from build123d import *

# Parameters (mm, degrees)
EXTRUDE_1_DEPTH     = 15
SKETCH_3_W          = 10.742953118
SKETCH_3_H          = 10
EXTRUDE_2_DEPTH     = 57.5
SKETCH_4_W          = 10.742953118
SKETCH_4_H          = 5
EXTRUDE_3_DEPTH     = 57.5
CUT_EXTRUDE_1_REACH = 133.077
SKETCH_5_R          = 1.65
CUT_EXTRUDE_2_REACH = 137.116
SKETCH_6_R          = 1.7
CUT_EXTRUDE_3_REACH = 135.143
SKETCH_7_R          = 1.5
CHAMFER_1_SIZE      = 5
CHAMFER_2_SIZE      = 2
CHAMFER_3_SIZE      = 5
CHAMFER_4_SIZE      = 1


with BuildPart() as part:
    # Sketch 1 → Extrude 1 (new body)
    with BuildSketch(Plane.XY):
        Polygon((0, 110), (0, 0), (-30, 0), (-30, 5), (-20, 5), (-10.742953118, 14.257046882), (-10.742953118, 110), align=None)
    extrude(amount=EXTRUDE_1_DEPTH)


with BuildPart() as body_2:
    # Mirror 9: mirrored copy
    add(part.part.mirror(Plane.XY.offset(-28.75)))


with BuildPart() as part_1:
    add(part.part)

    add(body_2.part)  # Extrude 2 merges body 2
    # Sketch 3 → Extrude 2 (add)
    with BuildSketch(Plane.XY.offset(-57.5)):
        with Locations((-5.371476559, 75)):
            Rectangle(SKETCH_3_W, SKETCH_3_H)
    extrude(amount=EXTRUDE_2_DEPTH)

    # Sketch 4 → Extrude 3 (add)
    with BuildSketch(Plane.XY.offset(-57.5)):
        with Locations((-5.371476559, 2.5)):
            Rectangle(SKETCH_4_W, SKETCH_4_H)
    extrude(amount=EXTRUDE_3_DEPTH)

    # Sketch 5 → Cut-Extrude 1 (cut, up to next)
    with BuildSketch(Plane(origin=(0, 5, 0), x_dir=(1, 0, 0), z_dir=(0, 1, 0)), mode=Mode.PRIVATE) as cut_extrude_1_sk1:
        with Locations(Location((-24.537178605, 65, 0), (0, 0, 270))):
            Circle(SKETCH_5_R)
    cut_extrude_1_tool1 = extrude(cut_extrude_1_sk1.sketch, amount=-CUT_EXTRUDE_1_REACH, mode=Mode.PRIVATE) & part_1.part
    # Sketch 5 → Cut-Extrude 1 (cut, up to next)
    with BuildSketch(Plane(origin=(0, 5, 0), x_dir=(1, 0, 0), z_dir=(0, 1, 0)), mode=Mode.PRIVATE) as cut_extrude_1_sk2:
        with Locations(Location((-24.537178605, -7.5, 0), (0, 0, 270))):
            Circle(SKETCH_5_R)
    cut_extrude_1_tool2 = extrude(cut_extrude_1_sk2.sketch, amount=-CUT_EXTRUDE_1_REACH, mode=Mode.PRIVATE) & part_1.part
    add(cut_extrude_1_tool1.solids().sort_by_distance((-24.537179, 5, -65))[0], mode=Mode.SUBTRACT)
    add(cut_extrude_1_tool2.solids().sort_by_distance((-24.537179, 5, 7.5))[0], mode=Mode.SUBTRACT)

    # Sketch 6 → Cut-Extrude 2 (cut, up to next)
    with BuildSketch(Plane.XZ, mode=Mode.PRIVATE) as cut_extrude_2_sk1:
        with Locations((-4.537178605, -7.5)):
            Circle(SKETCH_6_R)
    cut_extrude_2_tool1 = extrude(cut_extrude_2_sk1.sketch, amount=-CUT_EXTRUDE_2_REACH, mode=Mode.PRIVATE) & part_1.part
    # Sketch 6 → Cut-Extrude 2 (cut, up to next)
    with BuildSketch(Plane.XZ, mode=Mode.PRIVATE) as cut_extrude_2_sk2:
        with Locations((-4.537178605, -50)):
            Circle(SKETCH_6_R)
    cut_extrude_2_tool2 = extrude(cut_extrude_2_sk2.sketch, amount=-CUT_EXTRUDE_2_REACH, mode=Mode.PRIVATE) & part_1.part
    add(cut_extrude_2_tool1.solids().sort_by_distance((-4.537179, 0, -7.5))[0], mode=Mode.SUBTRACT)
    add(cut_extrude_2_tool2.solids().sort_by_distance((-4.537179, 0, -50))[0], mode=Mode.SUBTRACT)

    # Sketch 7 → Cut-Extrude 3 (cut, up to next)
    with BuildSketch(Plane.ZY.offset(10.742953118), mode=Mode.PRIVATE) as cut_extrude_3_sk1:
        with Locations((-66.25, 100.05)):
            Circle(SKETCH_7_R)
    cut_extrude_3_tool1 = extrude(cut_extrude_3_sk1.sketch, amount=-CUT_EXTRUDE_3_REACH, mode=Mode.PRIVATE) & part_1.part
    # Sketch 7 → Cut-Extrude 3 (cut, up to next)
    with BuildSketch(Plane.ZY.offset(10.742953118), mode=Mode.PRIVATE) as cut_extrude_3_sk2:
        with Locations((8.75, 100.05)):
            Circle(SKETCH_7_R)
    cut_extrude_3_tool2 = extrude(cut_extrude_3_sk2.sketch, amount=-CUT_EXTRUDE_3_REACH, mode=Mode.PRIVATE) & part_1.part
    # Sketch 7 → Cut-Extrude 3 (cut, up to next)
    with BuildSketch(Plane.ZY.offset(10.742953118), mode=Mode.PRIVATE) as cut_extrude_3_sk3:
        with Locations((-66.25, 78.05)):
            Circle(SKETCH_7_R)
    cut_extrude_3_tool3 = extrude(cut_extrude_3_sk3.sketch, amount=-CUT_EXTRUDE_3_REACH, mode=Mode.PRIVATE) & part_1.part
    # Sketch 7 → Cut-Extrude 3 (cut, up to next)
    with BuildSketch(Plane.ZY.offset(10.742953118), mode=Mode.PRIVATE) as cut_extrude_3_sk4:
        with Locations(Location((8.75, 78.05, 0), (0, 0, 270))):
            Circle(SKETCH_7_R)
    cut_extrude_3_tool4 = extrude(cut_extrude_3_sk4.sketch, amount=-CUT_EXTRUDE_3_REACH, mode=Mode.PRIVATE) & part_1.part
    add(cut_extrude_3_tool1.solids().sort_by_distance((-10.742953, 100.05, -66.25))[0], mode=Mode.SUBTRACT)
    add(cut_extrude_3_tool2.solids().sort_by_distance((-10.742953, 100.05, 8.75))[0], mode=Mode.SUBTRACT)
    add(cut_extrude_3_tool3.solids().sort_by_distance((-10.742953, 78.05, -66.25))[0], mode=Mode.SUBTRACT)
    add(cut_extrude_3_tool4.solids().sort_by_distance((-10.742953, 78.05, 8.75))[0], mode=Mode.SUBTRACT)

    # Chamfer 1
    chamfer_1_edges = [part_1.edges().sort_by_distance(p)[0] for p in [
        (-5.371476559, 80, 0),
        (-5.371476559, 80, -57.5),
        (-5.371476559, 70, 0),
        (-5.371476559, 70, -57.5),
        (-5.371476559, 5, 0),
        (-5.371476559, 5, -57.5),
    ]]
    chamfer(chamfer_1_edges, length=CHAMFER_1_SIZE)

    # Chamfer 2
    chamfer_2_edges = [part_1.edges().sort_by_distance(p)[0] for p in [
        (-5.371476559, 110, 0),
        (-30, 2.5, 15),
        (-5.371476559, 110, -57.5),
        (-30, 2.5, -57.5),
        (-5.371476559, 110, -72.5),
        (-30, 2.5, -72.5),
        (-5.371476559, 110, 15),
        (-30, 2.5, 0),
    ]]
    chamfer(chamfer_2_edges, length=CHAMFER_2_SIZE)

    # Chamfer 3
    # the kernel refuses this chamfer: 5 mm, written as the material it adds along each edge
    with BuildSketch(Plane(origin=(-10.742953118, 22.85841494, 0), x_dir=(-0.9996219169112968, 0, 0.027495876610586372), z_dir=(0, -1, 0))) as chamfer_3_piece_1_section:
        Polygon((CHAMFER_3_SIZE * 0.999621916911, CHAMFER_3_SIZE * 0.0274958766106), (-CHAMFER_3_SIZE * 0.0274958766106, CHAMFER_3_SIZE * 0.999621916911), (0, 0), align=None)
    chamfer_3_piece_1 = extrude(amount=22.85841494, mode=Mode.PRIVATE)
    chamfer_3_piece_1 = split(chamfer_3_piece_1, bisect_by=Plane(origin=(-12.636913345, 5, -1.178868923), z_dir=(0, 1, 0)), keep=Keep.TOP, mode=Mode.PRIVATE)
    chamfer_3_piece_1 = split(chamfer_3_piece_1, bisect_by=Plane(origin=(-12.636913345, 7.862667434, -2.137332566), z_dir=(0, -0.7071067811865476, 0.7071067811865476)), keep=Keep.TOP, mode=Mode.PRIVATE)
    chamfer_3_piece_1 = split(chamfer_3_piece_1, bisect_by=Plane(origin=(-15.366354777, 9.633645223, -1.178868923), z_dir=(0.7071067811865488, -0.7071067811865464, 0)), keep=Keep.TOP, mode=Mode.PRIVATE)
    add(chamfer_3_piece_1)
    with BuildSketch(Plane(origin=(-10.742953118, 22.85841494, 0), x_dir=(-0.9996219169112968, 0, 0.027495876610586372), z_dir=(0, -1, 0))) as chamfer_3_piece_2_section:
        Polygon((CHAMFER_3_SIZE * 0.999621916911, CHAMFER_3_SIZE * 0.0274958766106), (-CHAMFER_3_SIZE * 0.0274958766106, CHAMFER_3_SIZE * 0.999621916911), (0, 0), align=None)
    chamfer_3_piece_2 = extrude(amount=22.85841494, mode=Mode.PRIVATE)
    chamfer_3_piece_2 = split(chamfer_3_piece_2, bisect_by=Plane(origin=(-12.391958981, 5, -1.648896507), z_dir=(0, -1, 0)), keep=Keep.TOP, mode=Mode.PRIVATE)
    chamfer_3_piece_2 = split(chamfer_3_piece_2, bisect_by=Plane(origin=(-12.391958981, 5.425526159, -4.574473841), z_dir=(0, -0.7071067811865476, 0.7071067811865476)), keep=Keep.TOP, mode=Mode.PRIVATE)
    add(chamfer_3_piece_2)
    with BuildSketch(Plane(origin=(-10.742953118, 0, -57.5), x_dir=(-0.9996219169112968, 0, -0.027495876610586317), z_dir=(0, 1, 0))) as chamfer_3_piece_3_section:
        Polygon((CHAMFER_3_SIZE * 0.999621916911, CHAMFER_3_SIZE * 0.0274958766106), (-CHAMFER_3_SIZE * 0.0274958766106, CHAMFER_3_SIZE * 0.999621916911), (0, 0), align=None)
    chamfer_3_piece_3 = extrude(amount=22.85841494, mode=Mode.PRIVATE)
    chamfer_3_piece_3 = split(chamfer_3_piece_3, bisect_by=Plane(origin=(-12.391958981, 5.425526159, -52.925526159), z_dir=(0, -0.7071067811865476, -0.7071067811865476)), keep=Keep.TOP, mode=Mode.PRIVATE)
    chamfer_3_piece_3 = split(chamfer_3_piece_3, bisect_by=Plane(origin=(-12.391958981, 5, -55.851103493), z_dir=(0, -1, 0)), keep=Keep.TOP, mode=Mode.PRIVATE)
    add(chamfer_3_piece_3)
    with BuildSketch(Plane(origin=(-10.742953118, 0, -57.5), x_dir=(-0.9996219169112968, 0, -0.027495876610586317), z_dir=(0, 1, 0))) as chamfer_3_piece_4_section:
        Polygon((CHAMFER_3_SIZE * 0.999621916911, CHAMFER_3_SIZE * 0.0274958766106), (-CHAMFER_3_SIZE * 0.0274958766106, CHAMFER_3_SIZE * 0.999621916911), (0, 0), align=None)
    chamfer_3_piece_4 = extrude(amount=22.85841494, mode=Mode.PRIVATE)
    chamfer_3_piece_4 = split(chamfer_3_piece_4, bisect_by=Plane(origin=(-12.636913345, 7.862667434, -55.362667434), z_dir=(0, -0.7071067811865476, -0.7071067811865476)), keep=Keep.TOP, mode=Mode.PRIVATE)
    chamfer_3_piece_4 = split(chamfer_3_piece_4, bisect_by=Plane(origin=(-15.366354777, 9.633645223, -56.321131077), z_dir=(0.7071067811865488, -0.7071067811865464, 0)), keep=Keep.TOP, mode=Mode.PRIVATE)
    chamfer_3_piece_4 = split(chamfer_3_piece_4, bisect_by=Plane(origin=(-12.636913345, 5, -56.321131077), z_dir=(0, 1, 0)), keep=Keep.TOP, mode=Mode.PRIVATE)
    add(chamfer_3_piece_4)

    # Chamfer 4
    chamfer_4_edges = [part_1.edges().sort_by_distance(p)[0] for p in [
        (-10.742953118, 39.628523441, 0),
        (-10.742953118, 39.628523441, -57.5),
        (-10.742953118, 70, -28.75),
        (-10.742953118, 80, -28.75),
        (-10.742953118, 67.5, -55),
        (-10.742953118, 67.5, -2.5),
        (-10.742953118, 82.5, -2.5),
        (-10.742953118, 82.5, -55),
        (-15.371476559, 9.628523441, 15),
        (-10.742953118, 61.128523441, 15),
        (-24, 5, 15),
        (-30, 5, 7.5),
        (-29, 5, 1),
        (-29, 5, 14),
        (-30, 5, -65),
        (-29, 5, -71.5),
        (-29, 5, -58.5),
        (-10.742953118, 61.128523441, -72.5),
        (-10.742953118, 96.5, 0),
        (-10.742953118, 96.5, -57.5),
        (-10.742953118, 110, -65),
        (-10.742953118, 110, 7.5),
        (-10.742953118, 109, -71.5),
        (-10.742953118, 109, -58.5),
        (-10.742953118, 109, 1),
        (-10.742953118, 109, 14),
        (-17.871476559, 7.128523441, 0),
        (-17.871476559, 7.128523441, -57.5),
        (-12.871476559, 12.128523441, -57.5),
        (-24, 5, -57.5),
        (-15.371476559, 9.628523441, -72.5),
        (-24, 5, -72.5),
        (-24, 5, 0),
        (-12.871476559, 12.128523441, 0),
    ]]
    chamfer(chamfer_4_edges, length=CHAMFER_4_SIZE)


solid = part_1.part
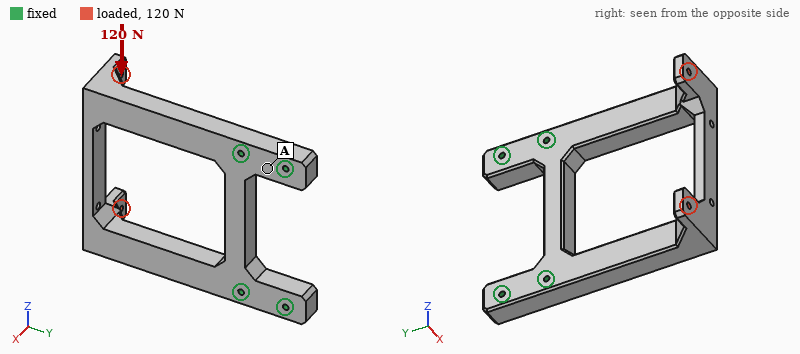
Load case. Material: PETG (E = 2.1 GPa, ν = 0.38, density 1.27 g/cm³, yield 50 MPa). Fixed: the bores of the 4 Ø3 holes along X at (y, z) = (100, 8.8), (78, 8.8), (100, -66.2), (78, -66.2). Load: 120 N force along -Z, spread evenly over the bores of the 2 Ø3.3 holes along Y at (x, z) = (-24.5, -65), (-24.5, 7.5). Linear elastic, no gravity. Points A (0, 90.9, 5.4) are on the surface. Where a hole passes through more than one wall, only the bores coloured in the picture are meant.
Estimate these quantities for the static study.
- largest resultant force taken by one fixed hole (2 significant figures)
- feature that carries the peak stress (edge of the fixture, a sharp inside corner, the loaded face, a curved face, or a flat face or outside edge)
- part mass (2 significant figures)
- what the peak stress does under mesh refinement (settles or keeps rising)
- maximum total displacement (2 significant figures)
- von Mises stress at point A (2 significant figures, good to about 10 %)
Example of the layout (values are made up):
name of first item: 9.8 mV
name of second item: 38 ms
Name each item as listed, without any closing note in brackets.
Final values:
largest resultant force taken by one fixed hole: 190 N
feature that carries the peak stress: a sharp inside corner
part mass: 62 g
what the peak stress does under mesh refinement: keeps rising
maximum total displacement: 1.7 mm
von Mises stress at point A: 1.9 MPa
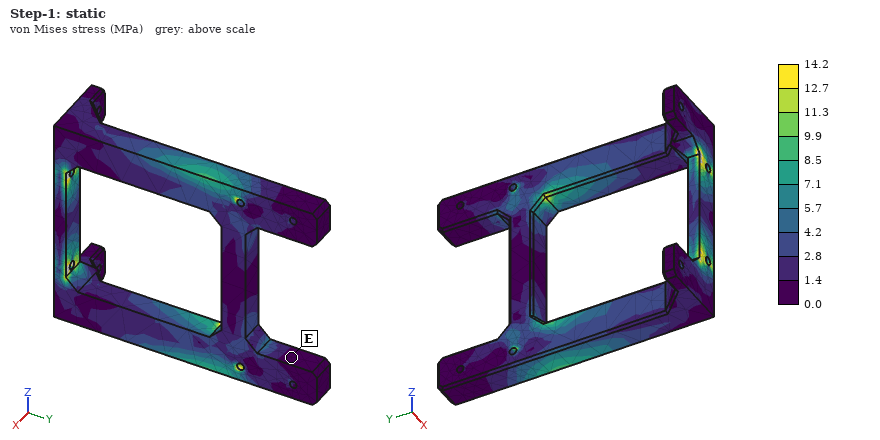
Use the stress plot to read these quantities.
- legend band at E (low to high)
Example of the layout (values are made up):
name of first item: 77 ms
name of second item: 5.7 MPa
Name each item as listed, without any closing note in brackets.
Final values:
legend band at E: 0.0 to 1.4 MPa
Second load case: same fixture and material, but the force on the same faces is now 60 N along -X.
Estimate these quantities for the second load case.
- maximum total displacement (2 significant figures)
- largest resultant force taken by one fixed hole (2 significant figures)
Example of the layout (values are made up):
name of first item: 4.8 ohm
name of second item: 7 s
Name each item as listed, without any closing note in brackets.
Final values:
maximum total displacement: 1.6 mm
largest resultant force taken by one fixed hole: 62 N
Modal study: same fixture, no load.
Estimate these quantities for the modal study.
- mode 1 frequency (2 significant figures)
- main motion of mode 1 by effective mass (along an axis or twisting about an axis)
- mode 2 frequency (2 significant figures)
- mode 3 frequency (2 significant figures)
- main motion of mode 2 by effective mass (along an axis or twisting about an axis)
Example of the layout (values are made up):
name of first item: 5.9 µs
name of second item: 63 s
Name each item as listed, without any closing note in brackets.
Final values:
mode 1 frequency: 250 Hz
main motion of mode 1 by effective mass: along X
mode 2 frequency: 380 Hz
mode 3 frequency: 420 Hz
main motion of mode 2 by effective mass: along Z
